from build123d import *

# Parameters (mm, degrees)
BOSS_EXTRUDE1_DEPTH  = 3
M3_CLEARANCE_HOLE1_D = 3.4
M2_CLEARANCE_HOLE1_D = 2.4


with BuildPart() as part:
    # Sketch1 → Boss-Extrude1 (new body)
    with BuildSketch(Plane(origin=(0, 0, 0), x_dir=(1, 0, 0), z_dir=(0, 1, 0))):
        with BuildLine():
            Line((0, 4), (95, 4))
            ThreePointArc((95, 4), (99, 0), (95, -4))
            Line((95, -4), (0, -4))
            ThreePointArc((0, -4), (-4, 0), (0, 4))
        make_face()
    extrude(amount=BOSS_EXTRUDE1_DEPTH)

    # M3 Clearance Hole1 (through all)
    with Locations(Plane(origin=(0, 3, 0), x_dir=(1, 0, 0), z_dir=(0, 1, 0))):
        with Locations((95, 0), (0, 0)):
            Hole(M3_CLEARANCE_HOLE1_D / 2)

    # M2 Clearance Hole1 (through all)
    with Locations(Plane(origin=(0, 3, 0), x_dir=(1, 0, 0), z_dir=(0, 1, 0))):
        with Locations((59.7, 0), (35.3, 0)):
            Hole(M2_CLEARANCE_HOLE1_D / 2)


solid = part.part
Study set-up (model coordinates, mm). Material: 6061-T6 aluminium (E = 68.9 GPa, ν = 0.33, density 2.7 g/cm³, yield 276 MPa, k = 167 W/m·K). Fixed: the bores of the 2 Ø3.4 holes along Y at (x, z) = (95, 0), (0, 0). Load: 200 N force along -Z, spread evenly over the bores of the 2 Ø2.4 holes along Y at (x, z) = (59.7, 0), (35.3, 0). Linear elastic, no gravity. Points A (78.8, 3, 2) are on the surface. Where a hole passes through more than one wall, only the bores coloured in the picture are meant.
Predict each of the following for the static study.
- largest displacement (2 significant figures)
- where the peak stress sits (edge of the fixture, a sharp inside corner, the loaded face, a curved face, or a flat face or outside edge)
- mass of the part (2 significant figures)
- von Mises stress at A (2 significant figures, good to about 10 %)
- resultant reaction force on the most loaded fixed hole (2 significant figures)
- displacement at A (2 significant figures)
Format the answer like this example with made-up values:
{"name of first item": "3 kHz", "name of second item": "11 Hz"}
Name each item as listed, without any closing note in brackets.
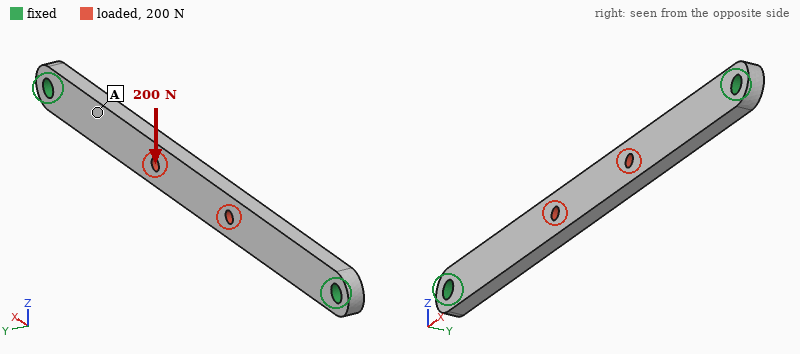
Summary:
{"largest displacement": "0.10 mm", "where the peak stress sits": "edge of the fixture", "mass of the part": "6.3 g", "von Mises stress at A": "12 MPa", "resultant reaction force on the most loaded fixed hole": "100 N", "displacement at A": "0.033 mm"}
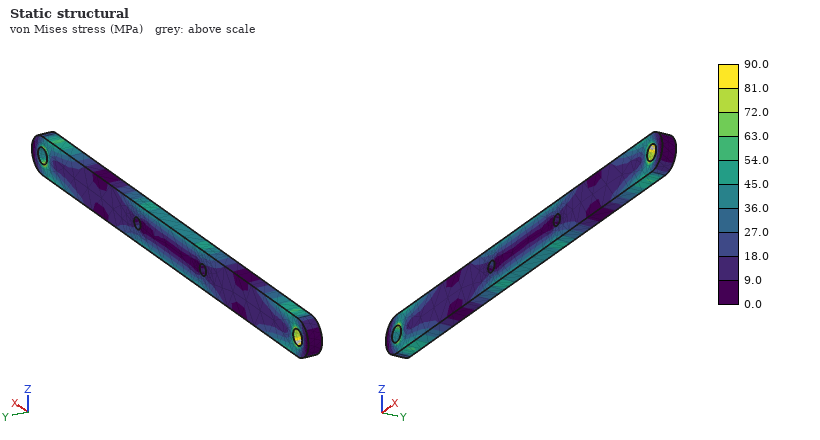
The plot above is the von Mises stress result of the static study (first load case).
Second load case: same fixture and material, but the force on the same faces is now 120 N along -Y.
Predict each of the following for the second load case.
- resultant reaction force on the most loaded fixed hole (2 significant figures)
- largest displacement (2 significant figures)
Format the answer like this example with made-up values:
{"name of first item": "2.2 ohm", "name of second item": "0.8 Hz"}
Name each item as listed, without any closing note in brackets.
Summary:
{"resultant reaction force on the most loaded fixed hole": "60 N", "largest displacement": "0.35 mm"}
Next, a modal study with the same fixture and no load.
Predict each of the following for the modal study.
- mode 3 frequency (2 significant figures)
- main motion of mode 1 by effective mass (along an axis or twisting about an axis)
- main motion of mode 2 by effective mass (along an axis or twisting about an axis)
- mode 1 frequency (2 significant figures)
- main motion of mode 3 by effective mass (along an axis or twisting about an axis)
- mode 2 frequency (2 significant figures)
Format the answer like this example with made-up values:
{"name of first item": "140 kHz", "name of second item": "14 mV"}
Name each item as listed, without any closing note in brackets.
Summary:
{"mode 3 frequency": "4800 Hz", "main motion of mode 1 by effective mass": "along Y", "main motion of mode 2 by effective mass": "along Z", "mode 1 frequency": "1800 Hz", "main motion of mode 3 by effective mass": "twisting about Z", "mode 2 frequency": "4200 Hz"}
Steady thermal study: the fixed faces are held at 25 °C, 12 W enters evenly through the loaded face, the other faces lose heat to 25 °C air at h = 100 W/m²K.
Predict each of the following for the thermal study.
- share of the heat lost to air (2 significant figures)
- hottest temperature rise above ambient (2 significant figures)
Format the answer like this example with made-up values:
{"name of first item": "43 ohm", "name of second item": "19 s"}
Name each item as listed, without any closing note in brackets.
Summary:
{"share of the heat lost to air": "37 %", "hottest temperature rise above ambient": "38 K"}
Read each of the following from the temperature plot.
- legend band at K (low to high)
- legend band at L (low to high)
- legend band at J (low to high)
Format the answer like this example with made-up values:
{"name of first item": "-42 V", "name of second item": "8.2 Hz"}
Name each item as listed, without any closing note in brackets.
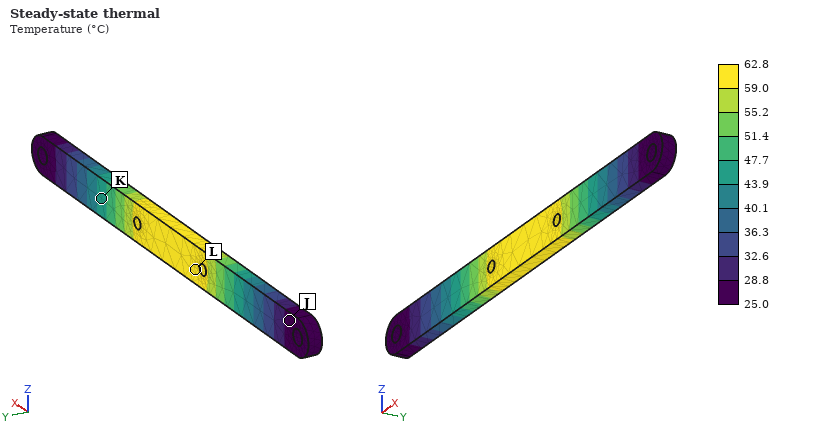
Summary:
{"legend band at K": "43.9 to 47.7 °C", "legend band at L": "59.0 to 62.8 °C", "legend band at J": "25.0 to 28.8 °C"}
